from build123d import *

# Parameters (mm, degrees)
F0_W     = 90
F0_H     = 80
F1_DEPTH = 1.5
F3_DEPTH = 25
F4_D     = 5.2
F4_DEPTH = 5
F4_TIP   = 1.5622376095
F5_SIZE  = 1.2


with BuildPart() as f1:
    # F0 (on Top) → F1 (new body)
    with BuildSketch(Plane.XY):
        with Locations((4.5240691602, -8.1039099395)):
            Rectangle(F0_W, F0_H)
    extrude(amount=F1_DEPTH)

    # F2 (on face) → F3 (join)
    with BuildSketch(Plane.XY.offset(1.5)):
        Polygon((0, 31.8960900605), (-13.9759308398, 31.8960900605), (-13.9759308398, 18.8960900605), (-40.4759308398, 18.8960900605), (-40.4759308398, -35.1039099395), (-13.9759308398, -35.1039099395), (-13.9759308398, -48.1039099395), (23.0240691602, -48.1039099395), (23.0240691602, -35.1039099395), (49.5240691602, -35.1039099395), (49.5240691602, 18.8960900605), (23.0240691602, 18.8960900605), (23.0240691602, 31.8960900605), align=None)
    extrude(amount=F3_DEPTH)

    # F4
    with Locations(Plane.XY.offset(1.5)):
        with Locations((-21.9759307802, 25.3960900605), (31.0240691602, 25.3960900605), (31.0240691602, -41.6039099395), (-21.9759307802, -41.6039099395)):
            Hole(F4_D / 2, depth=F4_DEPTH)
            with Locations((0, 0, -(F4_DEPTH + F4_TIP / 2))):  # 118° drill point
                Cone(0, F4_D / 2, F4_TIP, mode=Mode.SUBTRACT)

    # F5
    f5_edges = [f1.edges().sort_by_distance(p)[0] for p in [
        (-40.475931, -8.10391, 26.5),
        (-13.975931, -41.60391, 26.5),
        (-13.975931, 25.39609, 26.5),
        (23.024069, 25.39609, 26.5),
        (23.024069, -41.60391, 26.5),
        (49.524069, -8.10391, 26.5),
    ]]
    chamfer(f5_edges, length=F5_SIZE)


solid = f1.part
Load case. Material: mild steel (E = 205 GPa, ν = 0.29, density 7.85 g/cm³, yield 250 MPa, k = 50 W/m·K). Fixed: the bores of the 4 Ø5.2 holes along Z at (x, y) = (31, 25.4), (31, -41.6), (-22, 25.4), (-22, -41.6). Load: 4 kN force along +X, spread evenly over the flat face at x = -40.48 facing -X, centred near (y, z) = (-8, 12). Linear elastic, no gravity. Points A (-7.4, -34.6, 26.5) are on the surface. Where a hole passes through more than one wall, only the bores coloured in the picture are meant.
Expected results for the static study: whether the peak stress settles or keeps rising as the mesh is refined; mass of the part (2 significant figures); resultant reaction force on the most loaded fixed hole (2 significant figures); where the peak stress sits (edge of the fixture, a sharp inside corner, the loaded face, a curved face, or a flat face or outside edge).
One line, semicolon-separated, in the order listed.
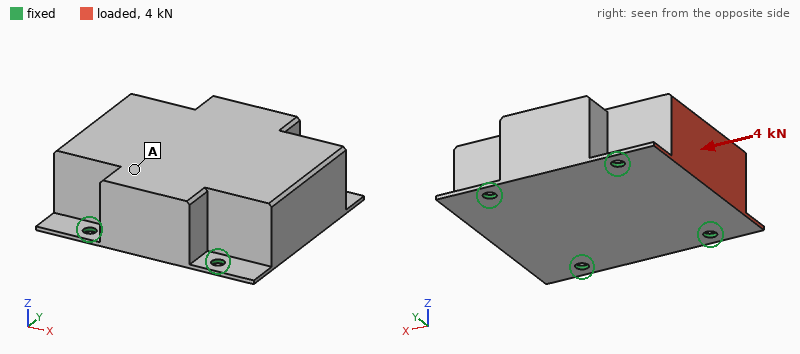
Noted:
keeps rising; 1.2 kg; 1.2 kN; edge of the fixture
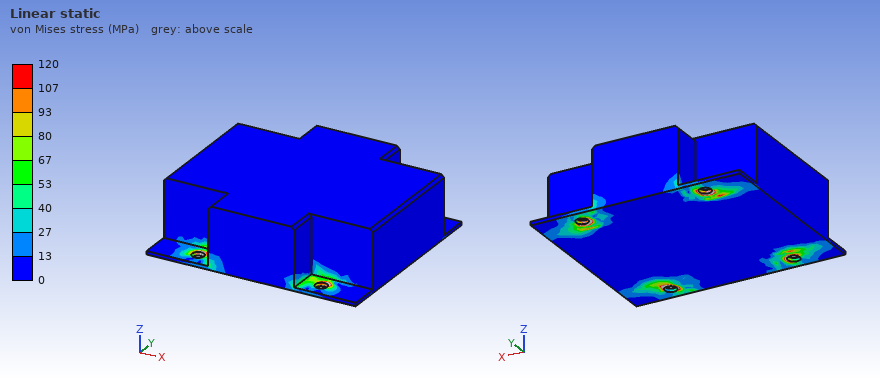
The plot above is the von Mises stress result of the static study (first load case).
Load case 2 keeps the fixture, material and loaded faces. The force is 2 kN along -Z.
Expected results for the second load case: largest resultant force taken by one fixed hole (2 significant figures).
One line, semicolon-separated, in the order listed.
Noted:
1.5 kN
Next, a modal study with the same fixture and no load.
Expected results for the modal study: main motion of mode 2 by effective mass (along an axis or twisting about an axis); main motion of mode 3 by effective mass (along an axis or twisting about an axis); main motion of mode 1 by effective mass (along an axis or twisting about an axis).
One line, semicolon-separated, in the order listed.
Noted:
along Z; along Y; along X
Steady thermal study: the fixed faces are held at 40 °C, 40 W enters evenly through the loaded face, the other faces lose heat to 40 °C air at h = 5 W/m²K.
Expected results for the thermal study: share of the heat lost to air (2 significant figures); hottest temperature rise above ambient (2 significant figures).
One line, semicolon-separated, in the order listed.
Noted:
9.5 %; 54 K
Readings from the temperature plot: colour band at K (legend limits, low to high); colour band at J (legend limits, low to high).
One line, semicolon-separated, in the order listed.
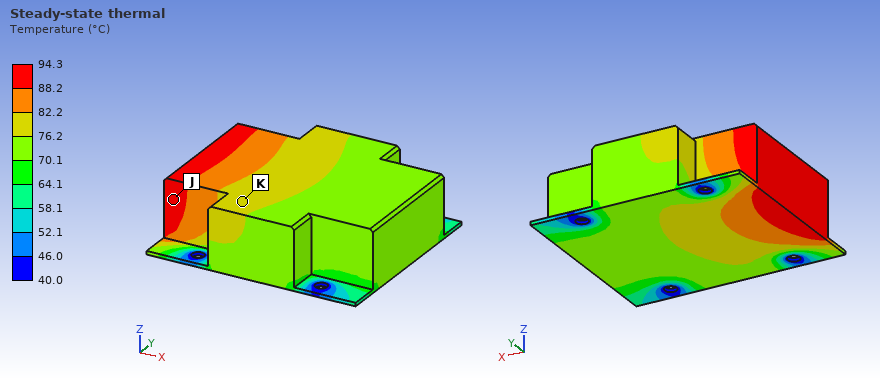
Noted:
76.2 to 82.2 °C; 88.2 to 94.3 °C
